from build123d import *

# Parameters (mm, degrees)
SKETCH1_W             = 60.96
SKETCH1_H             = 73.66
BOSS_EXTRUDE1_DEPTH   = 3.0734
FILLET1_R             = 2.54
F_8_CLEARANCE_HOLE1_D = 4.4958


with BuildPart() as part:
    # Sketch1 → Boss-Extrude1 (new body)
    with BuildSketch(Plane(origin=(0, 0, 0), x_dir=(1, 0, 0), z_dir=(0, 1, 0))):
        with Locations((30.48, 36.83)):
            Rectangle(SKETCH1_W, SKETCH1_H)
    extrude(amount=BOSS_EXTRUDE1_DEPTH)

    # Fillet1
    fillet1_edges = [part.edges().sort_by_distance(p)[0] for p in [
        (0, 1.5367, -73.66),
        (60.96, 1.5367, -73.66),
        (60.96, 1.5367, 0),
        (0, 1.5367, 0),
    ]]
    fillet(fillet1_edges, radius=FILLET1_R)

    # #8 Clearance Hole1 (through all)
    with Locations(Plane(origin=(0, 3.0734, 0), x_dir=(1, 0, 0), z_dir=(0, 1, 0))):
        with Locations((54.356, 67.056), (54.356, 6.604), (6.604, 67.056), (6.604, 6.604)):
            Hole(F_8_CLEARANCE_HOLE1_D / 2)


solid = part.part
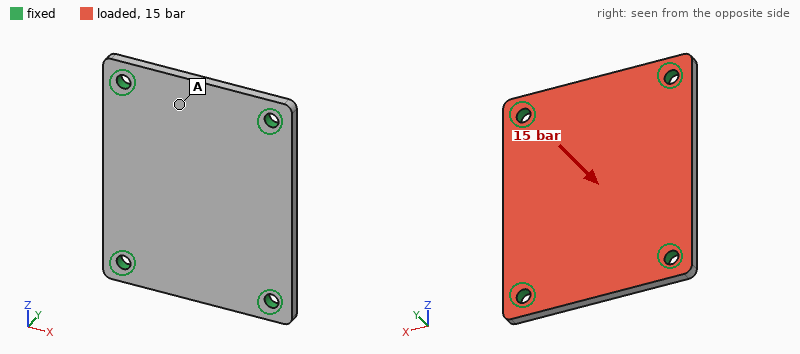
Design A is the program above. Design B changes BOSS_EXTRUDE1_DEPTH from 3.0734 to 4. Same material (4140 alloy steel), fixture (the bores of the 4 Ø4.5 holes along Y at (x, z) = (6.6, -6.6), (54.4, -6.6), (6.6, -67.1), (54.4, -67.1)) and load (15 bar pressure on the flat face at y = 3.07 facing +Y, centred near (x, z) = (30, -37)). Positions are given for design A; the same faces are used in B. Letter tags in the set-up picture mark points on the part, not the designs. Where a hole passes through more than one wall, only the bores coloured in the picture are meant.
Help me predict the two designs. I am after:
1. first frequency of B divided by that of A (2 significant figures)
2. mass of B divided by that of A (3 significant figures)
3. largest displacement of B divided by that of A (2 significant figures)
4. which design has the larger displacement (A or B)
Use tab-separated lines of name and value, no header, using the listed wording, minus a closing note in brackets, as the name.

first frequency of B divided by that of A	1.3
mass of B divided by that of A	1.30
largest displacement of B divided by that of A	0.48
which design has the larger displacement	A
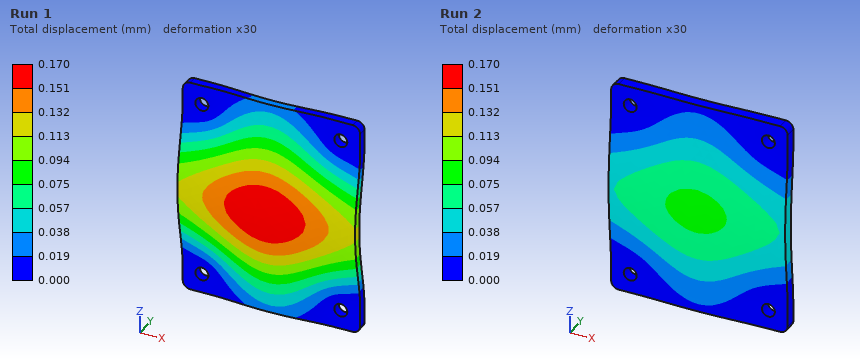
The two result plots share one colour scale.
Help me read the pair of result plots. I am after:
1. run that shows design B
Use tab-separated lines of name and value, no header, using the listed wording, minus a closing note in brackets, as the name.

run that shows design B	Run 2
